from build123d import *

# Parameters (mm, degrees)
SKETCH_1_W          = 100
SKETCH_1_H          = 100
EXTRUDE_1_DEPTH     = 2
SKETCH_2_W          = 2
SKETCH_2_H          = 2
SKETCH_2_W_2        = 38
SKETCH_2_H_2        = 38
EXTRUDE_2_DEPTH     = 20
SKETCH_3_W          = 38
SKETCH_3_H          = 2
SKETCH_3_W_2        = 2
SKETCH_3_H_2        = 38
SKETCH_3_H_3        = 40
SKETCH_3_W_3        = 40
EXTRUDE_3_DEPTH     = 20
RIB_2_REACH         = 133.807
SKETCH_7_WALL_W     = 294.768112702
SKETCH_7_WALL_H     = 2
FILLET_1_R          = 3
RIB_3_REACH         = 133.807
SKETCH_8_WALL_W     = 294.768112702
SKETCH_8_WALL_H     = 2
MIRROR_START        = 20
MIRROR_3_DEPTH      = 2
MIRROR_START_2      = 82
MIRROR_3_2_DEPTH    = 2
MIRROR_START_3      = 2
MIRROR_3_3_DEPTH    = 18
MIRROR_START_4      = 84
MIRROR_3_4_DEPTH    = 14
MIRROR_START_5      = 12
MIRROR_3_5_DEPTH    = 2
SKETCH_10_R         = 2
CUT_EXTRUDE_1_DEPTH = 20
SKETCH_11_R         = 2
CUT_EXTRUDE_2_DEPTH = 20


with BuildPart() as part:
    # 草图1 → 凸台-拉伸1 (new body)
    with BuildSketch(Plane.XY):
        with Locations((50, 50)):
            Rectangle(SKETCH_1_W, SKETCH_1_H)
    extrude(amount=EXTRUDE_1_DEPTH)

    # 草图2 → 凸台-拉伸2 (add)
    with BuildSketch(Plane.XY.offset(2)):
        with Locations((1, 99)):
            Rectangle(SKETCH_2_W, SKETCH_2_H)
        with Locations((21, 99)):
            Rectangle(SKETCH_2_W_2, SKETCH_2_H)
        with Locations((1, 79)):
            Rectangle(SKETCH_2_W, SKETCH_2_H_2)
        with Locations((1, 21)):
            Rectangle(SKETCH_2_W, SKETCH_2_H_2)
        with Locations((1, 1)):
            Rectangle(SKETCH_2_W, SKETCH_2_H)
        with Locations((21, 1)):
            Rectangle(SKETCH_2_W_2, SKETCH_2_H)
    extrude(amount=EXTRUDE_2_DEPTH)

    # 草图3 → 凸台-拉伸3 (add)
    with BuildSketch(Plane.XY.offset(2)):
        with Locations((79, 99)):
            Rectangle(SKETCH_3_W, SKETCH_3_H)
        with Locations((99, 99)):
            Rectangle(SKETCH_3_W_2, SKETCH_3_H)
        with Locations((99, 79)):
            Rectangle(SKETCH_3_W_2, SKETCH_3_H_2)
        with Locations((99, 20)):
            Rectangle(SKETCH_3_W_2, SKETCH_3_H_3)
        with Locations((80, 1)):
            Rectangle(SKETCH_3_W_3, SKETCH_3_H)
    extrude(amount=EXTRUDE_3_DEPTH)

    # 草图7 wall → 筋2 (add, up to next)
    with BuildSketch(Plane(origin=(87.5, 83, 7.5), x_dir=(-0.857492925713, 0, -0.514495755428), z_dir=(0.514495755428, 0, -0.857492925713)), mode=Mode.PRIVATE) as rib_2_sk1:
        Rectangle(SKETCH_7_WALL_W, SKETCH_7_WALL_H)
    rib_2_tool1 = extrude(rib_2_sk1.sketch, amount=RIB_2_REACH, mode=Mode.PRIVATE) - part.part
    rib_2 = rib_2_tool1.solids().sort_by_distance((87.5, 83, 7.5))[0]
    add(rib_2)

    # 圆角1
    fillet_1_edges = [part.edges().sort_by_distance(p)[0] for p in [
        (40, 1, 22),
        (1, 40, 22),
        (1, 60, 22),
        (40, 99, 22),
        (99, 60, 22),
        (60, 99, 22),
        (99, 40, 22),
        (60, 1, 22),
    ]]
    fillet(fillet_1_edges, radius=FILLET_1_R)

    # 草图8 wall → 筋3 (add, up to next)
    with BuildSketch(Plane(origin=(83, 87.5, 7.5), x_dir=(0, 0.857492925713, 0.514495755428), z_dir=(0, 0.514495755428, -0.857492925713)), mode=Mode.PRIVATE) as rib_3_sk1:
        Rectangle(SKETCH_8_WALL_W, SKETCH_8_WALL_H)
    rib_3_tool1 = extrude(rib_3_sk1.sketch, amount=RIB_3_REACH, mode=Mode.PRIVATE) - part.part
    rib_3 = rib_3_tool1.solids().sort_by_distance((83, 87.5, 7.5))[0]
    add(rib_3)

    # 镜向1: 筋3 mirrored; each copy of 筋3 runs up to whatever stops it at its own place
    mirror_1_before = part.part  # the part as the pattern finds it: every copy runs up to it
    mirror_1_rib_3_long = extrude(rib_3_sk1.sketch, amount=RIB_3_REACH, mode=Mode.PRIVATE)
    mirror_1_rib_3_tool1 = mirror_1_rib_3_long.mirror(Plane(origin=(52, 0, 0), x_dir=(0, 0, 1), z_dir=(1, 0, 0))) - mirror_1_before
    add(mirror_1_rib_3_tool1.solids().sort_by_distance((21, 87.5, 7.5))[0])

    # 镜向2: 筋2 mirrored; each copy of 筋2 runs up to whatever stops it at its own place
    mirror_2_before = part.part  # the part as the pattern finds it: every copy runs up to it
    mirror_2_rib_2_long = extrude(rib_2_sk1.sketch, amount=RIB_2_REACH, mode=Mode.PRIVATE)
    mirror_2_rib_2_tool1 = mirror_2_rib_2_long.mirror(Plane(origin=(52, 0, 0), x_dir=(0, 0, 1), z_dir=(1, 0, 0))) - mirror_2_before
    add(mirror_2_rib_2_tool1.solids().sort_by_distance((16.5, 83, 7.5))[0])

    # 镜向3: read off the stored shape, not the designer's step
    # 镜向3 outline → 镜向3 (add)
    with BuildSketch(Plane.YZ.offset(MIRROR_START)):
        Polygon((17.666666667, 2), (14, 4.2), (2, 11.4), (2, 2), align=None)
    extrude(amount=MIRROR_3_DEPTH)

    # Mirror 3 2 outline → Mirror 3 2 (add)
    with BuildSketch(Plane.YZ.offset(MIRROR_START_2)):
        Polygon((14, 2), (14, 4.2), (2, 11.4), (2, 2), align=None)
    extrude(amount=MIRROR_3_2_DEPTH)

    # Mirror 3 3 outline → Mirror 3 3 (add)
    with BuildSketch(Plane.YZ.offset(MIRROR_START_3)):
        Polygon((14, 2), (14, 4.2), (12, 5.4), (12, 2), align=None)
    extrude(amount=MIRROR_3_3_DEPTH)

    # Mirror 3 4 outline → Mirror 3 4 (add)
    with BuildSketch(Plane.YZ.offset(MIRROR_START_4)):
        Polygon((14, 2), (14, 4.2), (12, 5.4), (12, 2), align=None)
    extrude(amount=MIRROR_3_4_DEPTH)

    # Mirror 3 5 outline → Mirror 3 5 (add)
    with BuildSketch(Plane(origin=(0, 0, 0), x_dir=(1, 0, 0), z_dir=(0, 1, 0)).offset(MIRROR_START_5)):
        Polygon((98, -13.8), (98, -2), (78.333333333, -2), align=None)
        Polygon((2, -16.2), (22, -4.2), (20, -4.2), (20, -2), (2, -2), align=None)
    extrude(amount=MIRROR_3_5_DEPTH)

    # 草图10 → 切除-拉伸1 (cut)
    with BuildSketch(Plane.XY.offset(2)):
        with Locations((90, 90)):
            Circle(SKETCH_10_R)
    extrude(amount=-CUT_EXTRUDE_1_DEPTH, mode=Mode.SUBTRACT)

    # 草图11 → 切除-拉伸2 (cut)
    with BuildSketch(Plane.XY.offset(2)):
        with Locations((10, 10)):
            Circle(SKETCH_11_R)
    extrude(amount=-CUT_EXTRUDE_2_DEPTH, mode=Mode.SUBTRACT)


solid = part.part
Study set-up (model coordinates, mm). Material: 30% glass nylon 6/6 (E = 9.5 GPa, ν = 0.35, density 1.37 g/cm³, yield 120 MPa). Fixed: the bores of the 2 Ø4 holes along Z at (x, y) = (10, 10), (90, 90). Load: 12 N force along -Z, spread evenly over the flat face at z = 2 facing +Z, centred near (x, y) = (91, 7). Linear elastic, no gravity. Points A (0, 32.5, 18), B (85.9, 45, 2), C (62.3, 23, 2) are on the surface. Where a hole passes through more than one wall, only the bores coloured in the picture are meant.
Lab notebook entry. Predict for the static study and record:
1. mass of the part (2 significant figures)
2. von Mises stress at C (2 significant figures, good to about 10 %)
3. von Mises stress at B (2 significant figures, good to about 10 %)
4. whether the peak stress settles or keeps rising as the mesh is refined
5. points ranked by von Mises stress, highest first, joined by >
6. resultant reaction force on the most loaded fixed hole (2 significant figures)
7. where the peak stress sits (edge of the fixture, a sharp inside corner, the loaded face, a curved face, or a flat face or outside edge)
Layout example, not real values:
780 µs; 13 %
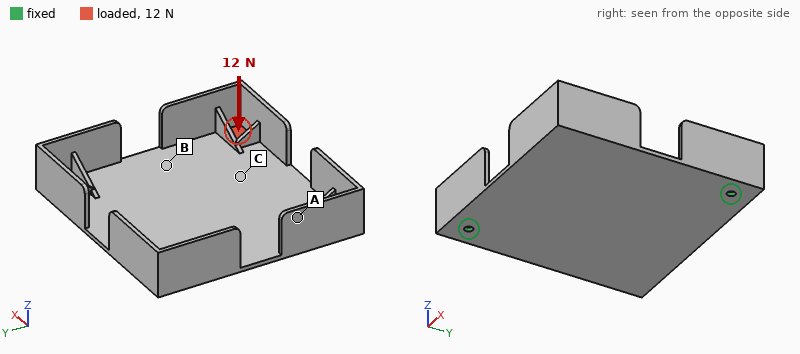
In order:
47 g; 5.2 MPa; 6.4 MPa; keeps rising; B > C > A; 8.1 N; edge of the fixture
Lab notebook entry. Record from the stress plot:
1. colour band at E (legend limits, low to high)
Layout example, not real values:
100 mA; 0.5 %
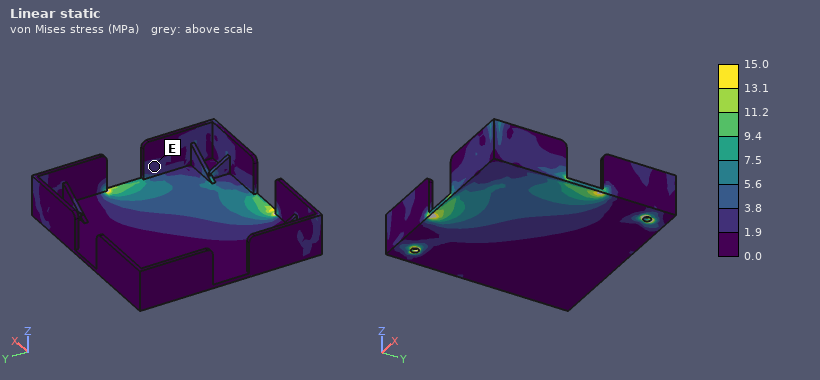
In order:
1.9 to 3.8 MPa
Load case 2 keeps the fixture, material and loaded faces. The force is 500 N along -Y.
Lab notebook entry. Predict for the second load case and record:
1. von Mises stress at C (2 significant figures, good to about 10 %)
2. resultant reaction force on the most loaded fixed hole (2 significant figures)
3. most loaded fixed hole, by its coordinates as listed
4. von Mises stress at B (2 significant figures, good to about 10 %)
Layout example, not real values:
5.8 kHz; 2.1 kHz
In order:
6.7 MPa; 420 N; (90, 90); 14 MPa
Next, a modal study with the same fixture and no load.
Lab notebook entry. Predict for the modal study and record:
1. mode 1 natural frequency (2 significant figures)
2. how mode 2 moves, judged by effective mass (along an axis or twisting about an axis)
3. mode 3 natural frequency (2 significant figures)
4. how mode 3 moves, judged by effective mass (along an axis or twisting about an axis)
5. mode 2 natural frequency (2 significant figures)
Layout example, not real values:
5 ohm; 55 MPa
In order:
190 Hz; along Z; 540 Hz; along Z; 220 Hz
